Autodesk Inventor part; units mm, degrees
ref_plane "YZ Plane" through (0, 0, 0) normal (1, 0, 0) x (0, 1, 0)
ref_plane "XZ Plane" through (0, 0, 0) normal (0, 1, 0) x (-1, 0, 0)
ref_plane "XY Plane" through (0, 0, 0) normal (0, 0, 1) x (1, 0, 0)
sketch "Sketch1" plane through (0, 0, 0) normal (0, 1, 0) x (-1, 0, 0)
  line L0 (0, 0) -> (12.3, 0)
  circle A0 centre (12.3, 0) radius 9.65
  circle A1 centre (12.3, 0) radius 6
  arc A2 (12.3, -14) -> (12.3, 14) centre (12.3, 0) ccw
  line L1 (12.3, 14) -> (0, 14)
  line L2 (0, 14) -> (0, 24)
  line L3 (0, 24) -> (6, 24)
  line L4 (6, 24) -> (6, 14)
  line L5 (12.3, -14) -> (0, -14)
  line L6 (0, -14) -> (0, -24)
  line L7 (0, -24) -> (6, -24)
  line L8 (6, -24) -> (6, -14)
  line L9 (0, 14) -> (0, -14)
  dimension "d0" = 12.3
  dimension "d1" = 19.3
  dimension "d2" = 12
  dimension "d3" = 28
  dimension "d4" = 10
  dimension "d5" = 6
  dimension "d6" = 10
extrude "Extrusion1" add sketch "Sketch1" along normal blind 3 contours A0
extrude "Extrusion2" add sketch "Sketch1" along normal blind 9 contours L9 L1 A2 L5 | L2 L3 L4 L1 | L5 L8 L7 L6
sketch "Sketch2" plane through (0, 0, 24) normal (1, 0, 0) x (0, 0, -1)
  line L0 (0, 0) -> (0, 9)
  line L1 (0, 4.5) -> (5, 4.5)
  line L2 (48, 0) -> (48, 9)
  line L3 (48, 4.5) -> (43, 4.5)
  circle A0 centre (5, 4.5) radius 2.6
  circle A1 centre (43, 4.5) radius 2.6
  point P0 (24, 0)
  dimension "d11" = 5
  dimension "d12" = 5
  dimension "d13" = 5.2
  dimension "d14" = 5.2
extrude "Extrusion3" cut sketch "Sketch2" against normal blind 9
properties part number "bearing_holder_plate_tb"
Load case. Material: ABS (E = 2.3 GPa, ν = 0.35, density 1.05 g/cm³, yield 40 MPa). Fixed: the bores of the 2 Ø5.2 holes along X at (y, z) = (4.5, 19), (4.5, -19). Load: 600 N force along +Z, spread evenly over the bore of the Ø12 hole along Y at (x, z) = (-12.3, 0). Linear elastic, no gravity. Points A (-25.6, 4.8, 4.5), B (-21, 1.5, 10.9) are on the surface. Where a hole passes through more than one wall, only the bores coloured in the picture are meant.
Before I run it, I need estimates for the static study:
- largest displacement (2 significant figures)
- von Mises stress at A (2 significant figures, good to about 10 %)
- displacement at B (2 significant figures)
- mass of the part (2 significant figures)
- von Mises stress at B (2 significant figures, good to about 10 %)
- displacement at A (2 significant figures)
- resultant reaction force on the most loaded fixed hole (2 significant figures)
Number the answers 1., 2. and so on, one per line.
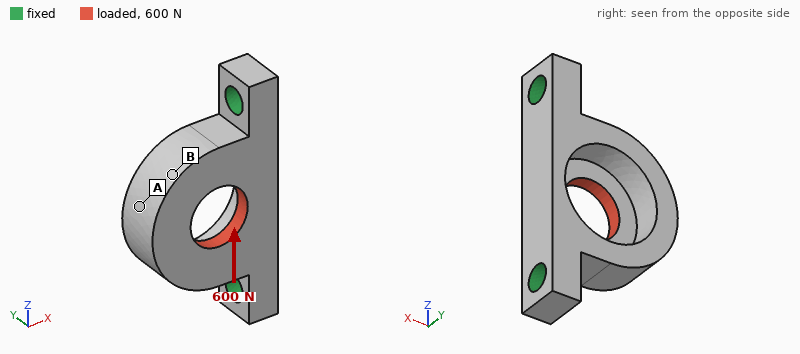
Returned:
1. 0.21 mm
2. 3.0 MPa
3. 0.19 mm
4. 4.8 g
5. 7.3 MPa
6. 0.18 mm
7. 350 N
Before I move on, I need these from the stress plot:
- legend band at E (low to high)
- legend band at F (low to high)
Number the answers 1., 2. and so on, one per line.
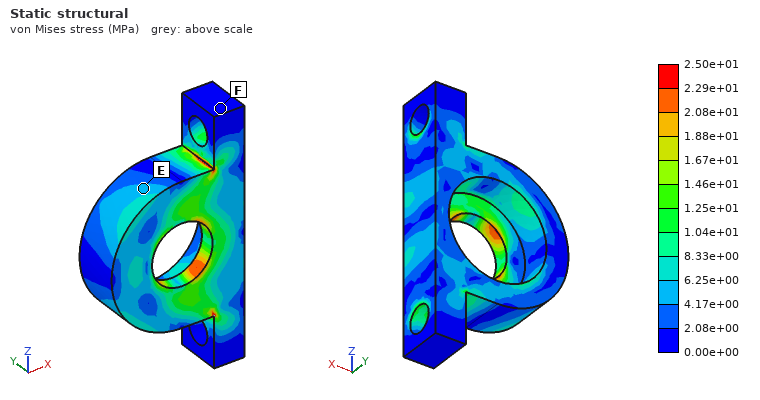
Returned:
1. 4.17e+00 to 6.25e+00 MPa
2. 0.00e+00 to 2.08e+00 MPa
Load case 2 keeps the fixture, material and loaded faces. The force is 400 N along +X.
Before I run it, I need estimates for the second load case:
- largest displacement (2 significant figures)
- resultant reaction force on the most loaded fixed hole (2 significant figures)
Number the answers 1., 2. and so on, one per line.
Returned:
1. 0.32 mm
2. 200 N
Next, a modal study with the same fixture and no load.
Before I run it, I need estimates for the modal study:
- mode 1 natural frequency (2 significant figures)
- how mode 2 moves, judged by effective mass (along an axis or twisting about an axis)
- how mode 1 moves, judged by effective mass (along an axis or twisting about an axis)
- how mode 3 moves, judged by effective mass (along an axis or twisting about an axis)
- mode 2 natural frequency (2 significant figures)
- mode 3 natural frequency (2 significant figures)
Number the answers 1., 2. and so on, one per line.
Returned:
1. 2000 Hz
2. along Z
3. along Y
4. along Z
5. 4400 Hz
6. 6000 Hz
